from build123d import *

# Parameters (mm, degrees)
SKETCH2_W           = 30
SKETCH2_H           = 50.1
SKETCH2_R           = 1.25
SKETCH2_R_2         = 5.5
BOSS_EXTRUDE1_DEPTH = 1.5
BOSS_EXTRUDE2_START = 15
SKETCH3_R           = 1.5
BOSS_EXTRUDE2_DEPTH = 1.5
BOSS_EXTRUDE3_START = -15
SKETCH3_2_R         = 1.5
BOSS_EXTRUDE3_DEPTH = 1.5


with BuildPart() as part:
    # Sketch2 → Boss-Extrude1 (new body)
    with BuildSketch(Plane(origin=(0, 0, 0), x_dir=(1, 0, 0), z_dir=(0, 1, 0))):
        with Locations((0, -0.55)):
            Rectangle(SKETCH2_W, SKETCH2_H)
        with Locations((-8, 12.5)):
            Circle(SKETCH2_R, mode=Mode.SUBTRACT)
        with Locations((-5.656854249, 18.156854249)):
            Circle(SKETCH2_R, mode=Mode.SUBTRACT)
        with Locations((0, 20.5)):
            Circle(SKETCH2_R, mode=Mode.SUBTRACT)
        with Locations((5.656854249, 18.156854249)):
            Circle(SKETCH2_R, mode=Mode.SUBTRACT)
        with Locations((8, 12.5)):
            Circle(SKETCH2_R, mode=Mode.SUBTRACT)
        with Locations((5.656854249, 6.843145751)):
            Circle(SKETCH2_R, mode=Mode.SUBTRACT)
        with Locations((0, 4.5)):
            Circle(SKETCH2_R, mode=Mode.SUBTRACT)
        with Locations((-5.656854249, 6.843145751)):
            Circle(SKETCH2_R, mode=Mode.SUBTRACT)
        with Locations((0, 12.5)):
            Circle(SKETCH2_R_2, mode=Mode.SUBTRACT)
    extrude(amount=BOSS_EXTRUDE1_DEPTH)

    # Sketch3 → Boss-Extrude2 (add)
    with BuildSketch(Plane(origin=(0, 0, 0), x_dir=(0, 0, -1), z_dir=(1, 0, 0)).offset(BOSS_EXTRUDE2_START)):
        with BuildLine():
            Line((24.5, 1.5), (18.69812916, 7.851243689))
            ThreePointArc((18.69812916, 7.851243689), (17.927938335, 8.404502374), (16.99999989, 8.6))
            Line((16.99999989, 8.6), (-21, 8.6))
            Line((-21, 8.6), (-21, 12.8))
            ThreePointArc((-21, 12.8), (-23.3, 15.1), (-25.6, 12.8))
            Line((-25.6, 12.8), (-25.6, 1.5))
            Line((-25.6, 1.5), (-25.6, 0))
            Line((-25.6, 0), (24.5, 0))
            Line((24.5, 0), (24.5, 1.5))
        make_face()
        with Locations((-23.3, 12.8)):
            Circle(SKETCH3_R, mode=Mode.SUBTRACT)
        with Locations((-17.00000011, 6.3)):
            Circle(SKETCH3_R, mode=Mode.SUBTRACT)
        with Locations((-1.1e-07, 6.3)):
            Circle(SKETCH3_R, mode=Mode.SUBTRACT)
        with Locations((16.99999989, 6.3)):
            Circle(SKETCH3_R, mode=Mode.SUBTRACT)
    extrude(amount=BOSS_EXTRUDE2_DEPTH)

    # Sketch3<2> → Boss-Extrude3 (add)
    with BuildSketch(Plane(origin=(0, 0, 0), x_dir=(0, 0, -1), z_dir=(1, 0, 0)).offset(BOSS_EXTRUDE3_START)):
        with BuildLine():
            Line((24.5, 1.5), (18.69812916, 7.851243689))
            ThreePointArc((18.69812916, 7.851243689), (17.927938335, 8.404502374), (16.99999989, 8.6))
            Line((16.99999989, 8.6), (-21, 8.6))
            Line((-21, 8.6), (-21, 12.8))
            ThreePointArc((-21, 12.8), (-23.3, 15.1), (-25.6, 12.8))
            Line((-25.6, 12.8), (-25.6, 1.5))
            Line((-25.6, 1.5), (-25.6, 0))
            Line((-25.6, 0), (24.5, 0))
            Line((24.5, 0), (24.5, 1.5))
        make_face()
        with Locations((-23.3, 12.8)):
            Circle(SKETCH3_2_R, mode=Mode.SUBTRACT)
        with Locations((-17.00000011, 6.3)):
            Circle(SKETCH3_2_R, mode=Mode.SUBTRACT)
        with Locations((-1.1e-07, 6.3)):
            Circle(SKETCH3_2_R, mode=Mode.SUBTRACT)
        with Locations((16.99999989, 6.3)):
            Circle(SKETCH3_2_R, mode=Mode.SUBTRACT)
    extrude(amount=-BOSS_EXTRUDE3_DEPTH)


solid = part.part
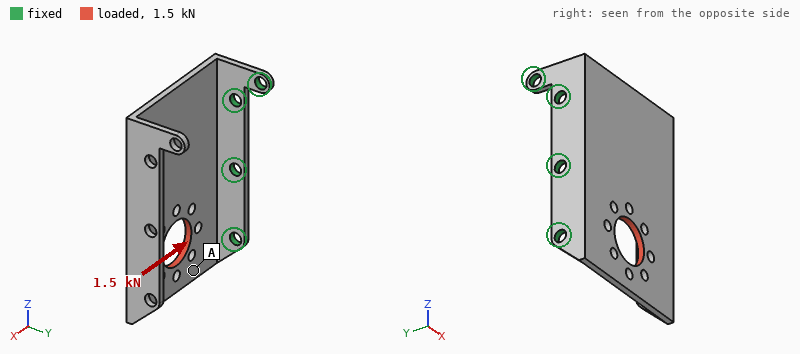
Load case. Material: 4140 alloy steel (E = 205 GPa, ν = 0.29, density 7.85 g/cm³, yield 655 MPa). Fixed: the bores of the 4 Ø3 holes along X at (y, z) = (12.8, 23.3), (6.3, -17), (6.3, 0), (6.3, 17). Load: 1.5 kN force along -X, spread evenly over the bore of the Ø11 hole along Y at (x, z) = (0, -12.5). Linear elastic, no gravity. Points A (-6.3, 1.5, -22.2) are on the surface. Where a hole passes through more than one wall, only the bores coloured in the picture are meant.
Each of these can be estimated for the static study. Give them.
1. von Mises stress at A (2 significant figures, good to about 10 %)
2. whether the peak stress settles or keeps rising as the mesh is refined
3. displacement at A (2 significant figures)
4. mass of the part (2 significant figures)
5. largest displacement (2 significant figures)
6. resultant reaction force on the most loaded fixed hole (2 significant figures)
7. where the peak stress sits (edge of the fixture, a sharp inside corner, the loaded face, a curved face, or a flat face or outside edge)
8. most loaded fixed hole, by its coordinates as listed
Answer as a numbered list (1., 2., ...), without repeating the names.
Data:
1. 100 MPa
2. keeps rising
3. 0.15 mm
4. 26 g
5. 0.36 mm
6. 1.0 kN
7. edge of the fixture
8. (6.3, -17)
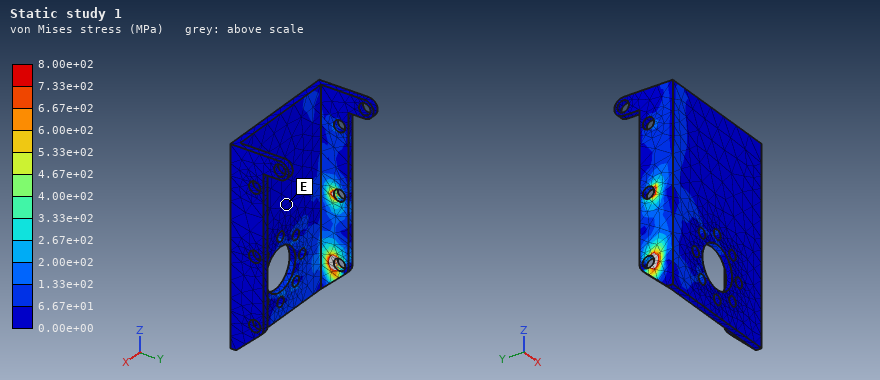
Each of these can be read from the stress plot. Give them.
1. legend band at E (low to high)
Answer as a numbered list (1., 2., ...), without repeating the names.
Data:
1. 0.00e+00 to 6.67e+01 MPa
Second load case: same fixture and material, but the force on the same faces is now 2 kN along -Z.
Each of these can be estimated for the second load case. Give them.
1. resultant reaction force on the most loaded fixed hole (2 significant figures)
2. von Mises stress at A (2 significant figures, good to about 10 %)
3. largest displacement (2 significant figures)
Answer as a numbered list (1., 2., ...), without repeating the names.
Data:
1. 1.1 kN
2. 130 MPa
3. 0.24 mm
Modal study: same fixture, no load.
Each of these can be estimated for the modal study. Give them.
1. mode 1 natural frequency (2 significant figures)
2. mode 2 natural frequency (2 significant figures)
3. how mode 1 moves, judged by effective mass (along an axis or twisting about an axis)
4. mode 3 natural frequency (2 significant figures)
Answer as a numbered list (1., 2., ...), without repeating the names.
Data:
1. 700 Hz
2. 1500 Hz
3. along Y
4. 4100 Hz
